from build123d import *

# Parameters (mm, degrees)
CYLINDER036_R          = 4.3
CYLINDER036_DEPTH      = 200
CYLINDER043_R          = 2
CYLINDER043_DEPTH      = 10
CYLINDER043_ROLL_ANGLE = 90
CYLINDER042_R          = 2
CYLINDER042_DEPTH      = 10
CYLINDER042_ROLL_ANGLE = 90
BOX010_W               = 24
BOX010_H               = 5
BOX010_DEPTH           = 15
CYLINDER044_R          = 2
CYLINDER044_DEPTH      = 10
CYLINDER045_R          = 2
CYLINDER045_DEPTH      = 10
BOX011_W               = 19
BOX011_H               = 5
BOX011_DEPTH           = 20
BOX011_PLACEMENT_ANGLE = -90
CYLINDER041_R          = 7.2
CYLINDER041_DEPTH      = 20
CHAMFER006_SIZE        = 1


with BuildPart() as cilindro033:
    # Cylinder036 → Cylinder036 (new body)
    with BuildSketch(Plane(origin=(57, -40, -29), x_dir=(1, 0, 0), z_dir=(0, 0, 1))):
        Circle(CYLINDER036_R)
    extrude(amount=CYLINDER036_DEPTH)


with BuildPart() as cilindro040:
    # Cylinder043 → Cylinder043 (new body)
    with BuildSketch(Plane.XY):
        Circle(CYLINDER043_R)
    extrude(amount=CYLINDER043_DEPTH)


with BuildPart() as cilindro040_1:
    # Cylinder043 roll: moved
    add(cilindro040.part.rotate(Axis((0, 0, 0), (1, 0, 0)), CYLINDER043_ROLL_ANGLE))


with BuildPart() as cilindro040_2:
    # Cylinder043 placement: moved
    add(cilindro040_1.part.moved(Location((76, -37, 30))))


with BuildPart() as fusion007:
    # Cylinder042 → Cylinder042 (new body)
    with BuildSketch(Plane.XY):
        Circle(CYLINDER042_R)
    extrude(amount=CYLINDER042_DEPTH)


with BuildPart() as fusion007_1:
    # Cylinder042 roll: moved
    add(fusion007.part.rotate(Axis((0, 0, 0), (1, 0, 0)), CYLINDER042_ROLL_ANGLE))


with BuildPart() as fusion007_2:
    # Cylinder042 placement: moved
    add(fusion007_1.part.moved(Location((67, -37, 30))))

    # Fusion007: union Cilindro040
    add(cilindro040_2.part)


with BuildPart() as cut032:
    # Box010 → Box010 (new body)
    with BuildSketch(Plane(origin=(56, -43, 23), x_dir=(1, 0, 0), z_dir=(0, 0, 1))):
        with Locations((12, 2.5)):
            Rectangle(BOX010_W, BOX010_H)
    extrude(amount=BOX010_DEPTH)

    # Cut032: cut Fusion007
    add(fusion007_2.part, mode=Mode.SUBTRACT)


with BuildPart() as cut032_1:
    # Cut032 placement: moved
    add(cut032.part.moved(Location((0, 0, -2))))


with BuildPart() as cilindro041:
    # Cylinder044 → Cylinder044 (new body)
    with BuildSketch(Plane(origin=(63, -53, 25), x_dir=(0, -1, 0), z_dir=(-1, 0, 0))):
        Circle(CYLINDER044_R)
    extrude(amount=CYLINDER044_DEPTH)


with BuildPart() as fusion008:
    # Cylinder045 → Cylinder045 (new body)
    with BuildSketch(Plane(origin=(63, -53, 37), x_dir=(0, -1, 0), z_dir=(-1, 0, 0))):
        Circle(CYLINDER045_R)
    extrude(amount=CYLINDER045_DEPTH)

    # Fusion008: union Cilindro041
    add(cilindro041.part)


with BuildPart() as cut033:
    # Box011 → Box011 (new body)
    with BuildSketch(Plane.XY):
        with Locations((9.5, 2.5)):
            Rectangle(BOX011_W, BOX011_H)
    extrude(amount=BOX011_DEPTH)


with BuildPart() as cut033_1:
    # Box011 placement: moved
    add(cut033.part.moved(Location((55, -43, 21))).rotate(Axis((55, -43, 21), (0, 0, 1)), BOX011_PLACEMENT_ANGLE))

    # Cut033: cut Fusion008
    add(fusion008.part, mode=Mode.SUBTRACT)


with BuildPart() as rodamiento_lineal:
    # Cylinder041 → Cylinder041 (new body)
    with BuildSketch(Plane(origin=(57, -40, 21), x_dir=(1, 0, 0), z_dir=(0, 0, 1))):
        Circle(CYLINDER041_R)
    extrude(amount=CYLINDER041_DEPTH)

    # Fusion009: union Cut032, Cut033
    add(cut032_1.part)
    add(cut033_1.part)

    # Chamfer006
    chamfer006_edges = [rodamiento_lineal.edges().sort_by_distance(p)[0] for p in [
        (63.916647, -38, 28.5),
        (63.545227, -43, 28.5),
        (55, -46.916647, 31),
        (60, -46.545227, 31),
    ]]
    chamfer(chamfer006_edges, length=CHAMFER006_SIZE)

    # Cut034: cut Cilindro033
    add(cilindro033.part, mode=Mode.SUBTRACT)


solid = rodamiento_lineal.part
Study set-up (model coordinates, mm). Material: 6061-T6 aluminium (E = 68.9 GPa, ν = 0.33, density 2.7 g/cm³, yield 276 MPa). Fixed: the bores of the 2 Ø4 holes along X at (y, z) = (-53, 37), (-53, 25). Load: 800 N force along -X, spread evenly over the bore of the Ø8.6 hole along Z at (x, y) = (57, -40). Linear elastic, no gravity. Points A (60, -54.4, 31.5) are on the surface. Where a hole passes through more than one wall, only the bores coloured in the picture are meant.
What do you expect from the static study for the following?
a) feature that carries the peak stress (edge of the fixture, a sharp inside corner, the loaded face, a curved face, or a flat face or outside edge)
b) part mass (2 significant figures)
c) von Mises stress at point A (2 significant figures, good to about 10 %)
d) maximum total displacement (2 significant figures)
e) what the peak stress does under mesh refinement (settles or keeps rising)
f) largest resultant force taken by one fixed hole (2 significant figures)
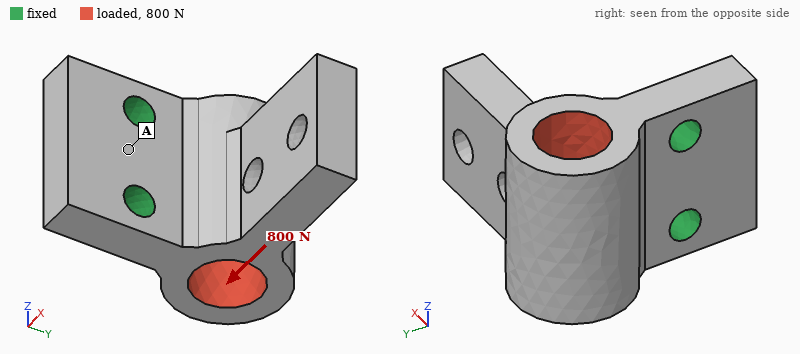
edge of the fixture
12 g
24 MPa
0.12 mm
keeps rising
400 N
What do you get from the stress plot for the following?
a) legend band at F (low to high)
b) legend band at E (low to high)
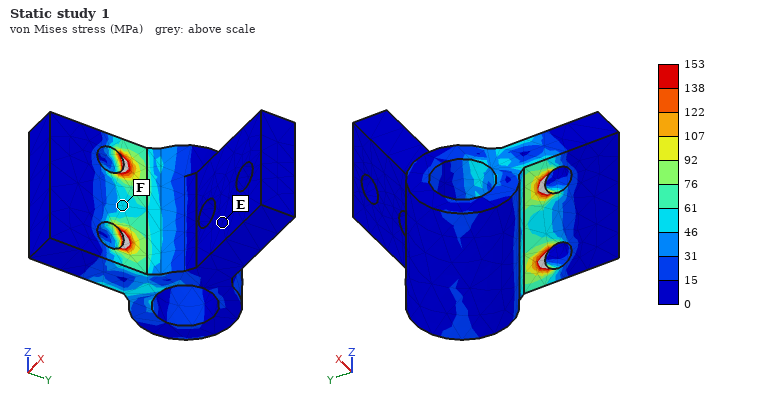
46 to 61 MPa
0 to 15 MPa
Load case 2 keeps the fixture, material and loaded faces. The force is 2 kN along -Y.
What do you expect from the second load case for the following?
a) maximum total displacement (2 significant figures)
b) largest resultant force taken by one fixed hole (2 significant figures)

13 µm
1.0 kN
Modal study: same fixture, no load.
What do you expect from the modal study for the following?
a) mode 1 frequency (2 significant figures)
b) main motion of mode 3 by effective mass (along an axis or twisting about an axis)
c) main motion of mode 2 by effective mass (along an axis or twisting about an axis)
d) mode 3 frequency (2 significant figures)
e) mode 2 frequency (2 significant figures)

4800 Hz
along X
along Z
15 kHz
11 kHz
